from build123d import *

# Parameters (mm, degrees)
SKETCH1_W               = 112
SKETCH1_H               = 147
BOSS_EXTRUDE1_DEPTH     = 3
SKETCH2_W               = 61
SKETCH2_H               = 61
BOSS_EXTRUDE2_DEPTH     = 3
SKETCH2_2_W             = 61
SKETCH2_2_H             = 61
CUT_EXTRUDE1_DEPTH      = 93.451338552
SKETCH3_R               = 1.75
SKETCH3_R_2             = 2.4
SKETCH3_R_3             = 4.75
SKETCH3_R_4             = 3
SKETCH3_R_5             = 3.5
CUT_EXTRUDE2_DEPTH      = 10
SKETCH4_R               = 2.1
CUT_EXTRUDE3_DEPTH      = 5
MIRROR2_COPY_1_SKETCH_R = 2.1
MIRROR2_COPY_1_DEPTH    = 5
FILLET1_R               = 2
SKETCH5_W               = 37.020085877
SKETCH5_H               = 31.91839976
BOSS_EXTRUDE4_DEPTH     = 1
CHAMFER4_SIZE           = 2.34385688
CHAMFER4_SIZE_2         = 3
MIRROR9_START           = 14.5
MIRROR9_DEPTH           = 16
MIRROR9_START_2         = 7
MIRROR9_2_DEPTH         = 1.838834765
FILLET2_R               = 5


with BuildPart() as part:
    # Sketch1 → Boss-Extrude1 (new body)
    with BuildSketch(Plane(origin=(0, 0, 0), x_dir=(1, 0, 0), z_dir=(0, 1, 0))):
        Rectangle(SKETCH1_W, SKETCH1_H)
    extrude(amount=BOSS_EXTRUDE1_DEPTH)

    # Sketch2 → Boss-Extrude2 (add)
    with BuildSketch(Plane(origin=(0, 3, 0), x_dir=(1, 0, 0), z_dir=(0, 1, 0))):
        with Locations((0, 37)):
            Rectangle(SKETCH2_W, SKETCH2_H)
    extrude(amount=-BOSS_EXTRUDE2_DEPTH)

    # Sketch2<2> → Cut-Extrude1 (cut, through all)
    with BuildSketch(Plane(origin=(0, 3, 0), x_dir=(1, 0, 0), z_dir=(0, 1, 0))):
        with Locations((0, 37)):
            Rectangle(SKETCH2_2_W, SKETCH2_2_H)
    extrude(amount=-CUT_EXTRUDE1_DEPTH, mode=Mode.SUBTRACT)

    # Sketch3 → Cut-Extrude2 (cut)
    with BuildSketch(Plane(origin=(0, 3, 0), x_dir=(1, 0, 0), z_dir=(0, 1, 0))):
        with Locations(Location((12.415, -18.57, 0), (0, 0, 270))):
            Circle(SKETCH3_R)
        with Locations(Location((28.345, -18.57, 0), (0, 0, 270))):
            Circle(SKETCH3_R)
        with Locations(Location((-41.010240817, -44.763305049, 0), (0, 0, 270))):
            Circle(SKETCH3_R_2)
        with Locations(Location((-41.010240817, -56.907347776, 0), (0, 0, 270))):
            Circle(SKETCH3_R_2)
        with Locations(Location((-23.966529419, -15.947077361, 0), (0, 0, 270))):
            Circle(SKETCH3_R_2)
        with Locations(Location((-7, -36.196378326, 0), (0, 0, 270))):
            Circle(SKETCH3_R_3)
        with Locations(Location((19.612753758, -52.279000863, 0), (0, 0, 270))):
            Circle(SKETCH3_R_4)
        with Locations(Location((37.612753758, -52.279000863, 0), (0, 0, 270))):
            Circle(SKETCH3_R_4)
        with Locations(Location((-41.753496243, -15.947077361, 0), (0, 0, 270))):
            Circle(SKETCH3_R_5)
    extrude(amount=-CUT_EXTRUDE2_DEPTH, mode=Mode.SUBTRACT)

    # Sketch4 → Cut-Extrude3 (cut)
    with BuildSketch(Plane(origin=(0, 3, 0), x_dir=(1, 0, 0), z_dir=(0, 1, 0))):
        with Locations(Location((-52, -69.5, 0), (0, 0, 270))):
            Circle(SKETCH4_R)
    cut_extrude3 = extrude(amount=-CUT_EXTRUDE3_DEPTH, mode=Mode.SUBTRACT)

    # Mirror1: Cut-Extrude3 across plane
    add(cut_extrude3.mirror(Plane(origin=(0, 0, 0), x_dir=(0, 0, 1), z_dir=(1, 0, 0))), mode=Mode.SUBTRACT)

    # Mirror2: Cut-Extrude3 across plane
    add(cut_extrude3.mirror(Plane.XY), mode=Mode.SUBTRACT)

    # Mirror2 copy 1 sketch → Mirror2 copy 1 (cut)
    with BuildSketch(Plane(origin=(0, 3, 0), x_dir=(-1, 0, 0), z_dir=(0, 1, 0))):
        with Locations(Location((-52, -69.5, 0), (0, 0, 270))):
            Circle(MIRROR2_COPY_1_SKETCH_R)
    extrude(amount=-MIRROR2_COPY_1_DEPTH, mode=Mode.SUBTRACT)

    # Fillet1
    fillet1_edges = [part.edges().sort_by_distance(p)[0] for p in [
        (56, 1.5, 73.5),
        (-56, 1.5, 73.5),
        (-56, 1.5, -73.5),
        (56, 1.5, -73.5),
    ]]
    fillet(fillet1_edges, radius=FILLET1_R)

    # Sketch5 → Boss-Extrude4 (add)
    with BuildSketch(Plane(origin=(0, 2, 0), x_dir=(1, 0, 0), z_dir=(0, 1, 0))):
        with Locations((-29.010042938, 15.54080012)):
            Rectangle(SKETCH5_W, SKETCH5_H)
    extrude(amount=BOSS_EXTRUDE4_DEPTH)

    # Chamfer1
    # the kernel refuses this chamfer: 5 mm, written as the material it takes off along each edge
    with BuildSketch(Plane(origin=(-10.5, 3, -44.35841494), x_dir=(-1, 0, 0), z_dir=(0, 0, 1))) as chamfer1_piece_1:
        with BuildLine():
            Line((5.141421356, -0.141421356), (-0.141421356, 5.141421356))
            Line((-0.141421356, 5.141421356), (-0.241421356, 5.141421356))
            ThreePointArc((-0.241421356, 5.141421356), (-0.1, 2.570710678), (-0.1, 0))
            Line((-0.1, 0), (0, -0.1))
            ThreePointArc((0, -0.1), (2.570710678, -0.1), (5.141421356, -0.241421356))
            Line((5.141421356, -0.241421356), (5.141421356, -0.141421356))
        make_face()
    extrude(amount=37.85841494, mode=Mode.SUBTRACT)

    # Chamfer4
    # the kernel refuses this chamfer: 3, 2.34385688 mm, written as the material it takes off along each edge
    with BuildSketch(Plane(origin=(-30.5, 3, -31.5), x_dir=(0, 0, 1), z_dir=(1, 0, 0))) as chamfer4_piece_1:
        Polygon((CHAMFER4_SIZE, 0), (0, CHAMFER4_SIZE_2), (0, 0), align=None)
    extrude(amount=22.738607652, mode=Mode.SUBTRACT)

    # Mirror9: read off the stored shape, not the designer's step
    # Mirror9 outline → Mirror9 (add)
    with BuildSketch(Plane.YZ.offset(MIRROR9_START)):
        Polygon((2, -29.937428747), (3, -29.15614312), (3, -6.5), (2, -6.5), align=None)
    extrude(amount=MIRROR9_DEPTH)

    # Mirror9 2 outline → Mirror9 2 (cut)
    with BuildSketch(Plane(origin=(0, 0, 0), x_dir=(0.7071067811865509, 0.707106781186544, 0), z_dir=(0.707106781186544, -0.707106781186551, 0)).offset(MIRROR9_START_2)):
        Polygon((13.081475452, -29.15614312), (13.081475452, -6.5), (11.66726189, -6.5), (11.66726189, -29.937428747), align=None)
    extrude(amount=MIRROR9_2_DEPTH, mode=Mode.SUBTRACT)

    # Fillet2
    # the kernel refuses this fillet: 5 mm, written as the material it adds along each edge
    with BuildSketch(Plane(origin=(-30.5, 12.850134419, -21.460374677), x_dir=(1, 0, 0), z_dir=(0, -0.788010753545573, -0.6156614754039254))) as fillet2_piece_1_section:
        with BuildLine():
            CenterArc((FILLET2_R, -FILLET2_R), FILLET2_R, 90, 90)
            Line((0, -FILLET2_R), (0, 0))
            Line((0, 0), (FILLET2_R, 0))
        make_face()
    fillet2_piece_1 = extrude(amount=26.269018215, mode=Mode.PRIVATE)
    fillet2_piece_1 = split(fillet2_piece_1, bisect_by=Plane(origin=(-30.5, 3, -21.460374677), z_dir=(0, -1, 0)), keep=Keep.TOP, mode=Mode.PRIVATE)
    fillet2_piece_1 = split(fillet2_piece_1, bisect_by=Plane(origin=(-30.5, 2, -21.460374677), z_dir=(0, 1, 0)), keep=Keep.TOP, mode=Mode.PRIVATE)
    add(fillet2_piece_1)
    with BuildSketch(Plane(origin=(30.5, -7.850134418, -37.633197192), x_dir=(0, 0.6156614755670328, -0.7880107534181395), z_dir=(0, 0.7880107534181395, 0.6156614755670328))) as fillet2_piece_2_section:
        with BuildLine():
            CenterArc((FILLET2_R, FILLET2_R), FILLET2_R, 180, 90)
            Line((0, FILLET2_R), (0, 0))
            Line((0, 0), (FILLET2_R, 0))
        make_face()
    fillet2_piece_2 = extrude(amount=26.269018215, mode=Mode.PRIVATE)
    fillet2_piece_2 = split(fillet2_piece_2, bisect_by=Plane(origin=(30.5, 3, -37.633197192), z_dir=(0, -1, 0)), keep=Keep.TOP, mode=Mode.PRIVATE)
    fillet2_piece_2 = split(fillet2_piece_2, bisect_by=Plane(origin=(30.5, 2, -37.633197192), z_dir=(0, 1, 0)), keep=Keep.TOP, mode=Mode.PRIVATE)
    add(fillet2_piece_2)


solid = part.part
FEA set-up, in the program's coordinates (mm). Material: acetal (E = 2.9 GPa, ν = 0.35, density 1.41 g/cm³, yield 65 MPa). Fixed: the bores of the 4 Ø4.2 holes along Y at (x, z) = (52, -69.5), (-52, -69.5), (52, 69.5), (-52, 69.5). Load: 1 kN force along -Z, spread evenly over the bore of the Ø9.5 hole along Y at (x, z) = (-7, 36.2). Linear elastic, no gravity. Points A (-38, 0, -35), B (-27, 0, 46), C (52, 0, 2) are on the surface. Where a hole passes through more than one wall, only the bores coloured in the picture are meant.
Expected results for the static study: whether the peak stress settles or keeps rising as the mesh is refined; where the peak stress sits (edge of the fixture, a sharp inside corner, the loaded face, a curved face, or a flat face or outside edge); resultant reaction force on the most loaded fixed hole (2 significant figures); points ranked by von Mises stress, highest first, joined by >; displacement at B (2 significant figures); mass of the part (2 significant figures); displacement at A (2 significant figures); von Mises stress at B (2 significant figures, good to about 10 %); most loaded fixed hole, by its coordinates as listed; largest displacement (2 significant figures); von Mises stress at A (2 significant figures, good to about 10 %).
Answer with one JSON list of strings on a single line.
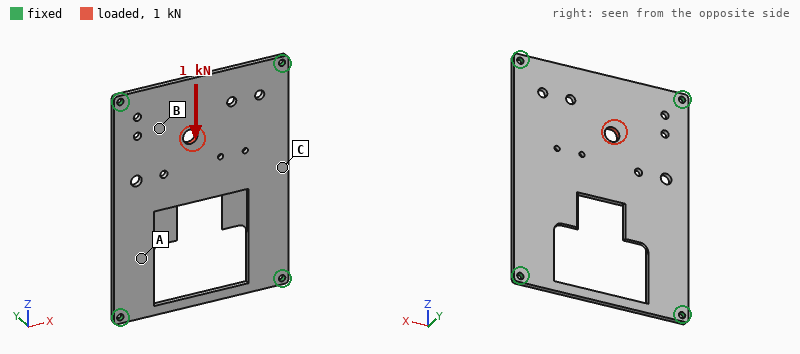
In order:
["keeps rising", "edge of the fixture", "400 N", "B > A > C", "0.13 mm", "54 g", "0.086 mm", "5.2 MPa", "(-52, 69.5)", "0.25 mm", "2.8 MPa"]
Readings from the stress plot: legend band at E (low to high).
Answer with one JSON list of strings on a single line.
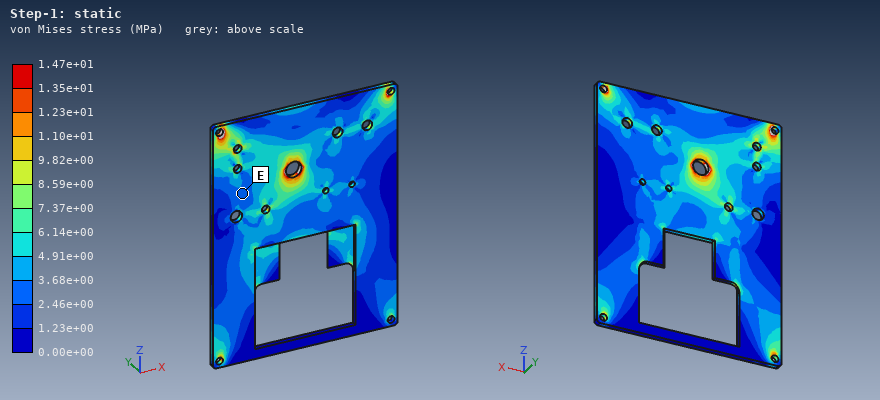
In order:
["2.46e+00 to 3.68e+00 MPa"]
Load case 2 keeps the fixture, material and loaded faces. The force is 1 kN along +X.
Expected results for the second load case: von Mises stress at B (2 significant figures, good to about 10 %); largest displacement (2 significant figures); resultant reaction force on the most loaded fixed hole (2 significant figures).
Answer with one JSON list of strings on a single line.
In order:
["6.6 MPa", "0.22 mm", "540 N"]
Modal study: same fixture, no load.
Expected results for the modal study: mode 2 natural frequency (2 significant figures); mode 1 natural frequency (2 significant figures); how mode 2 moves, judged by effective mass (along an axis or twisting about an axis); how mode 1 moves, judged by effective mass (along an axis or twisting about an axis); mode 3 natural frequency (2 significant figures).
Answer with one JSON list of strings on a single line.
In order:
["260 Hz", "160 Hz", "twisting about Z", "along Y", "380 Hz"]
